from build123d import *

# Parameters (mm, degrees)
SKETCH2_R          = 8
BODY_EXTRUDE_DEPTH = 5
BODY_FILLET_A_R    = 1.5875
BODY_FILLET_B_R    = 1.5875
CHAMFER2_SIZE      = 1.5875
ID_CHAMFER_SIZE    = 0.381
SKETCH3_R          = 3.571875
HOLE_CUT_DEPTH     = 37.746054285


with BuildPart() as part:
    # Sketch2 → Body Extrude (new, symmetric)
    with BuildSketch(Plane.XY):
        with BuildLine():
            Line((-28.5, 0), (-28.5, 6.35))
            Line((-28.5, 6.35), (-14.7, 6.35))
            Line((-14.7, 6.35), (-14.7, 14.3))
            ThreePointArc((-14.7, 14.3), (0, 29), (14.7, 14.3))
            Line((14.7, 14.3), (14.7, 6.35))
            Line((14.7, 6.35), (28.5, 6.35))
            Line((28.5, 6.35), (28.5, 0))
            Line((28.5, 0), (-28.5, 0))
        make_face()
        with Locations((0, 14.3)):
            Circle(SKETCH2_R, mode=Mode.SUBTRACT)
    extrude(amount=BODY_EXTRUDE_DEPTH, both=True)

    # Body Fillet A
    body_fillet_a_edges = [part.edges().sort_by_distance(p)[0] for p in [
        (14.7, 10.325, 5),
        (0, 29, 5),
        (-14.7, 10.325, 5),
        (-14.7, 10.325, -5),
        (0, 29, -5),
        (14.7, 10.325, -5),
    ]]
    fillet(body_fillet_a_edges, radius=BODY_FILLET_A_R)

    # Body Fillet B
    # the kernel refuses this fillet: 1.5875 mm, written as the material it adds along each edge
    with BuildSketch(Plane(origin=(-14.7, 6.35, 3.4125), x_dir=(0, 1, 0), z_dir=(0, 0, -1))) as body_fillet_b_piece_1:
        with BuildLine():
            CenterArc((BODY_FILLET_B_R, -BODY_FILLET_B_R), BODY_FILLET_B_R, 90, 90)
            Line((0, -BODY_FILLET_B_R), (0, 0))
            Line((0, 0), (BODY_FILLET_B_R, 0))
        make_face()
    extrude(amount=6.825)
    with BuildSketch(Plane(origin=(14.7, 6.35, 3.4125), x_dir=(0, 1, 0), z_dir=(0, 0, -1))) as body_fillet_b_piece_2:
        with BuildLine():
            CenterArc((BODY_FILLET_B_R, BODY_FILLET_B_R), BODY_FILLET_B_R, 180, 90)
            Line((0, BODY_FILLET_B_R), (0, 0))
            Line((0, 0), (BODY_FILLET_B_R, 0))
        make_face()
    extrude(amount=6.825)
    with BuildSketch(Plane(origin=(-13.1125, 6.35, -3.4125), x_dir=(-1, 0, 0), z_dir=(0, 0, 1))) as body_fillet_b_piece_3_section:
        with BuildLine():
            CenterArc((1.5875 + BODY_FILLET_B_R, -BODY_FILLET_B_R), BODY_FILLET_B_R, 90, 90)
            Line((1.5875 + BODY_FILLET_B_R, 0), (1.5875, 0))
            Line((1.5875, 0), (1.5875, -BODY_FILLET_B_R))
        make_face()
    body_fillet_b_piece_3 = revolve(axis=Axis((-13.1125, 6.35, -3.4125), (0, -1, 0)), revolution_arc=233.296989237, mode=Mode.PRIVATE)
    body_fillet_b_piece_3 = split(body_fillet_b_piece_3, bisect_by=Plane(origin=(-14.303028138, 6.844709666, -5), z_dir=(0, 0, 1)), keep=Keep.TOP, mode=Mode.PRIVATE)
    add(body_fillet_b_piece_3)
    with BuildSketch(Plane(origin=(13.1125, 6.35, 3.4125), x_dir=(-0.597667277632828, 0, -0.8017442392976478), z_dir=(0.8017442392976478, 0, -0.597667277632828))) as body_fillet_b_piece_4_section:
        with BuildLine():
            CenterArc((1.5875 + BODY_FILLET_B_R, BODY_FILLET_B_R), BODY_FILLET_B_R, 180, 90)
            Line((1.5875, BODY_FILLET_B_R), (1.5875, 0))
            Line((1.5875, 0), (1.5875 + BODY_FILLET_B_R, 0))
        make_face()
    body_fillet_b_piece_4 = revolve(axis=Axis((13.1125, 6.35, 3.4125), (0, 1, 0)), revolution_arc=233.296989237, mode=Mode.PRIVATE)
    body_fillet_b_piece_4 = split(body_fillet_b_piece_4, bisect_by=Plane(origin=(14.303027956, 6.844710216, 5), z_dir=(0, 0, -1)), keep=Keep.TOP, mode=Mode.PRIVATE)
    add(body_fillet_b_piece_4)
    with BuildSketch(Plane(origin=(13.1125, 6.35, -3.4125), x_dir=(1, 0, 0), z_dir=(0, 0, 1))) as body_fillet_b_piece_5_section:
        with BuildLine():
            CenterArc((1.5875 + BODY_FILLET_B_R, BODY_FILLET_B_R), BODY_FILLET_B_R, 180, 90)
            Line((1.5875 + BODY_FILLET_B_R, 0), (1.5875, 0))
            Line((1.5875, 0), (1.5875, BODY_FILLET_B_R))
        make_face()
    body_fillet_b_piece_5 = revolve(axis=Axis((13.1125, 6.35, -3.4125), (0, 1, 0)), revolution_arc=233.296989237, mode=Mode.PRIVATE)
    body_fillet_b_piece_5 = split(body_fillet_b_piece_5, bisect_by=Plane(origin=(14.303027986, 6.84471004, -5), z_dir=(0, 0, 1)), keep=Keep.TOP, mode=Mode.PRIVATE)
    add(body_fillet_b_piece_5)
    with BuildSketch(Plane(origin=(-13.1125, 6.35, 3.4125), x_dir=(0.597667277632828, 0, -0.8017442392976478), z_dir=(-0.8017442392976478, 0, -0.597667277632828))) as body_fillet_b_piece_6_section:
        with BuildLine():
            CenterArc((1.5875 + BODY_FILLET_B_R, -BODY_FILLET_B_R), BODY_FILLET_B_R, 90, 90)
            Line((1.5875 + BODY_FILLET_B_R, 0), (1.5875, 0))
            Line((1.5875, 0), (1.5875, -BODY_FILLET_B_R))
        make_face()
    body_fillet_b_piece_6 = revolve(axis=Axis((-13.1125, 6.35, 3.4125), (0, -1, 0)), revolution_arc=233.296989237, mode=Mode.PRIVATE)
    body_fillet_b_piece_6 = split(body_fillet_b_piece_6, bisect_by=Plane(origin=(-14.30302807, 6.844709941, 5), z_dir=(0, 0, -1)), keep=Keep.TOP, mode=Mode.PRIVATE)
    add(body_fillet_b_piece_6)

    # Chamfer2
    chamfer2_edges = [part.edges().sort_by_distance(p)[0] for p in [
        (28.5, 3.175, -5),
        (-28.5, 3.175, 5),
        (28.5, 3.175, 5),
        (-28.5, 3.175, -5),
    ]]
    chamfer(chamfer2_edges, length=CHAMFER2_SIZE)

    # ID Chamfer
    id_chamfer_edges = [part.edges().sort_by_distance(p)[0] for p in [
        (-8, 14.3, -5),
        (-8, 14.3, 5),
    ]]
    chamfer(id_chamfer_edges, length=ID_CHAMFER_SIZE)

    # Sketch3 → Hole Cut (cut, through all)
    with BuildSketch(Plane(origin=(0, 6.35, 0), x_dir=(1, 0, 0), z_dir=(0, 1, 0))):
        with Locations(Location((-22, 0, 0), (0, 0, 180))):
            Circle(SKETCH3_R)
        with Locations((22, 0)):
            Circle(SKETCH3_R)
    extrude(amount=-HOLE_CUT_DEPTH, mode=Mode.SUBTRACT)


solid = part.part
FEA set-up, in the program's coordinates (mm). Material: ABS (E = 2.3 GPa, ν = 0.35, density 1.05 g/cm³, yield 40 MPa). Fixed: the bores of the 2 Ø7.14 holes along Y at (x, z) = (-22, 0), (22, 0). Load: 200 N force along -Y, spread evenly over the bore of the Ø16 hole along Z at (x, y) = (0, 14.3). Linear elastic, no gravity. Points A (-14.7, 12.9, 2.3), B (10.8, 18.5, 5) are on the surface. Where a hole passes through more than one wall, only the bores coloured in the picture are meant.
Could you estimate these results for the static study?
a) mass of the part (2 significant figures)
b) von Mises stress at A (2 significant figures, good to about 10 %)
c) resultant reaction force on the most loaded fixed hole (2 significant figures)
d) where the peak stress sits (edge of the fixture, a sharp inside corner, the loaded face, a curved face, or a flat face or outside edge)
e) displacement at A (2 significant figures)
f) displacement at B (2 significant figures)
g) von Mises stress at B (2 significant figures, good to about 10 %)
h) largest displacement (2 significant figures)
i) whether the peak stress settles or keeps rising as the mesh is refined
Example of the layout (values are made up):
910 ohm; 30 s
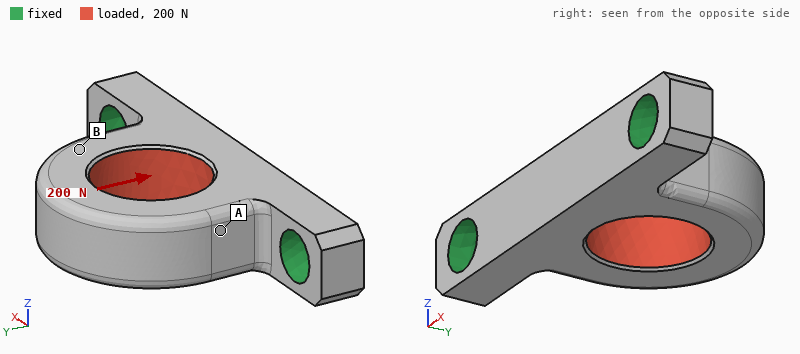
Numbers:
7.1 g; 2.3 MPa; 110 N; edge of the fixture; 28 µm; 30 µm; 1.1 MPa; 42 µm; keeps rising
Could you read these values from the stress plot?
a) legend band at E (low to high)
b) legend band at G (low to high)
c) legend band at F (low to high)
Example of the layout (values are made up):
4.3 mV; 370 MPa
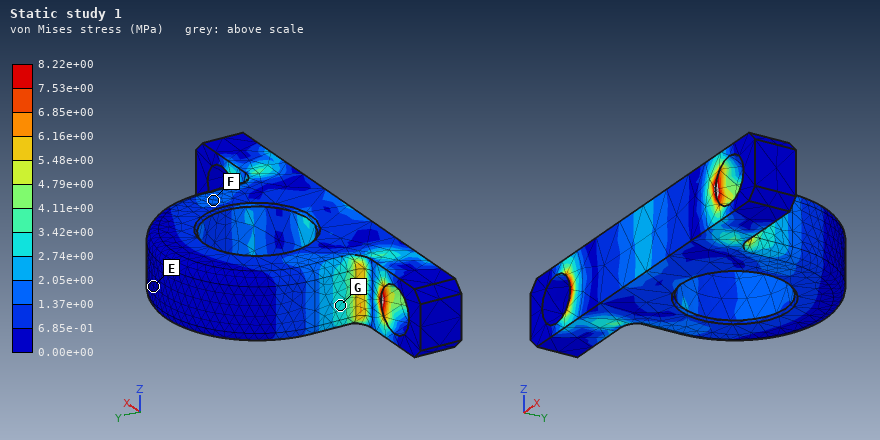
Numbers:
0.00e+00 to 6.85e-01 MPa; 2.74e+00 to 3.42e+00 MPa; 1.37e+00 to 2.05e+00 MPa
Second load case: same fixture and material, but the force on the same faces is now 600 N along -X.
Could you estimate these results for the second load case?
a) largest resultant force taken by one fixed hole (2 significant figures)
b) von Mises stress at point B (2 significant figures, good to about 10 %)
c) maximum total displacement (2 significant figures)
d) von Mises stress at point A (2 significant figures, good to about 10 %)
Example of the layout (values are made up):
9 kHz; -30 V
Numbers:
350 N; 3.6 MPa; 0.18 mm; 3.7 MPa
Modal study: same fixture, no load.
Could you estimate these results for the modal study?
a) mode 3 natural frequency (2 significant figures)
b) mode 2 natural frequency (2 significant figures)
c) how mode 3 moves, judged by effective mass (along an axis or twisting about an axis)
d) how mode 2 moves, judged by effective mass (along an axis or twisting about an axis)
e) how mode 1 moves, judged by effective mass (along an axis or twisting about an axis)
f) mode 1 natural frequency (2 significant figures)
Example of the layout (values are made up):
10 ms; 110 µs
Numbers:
5200 Hz; 4600 Hz; twisting about Y; along X; along Z; 1700 Hz
